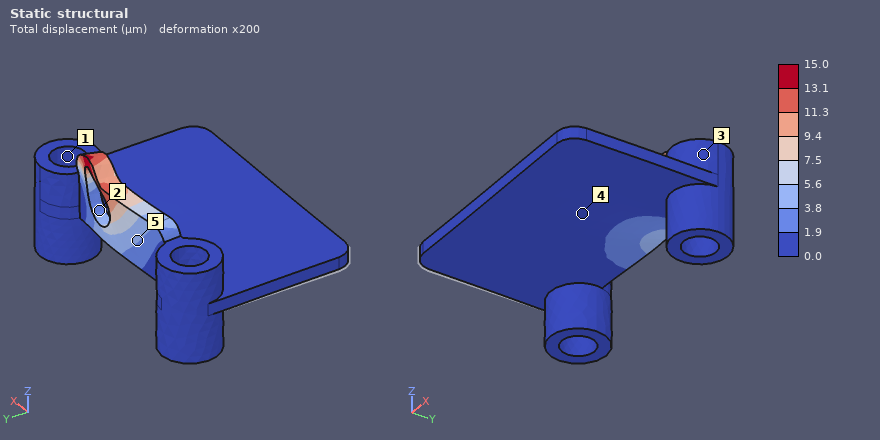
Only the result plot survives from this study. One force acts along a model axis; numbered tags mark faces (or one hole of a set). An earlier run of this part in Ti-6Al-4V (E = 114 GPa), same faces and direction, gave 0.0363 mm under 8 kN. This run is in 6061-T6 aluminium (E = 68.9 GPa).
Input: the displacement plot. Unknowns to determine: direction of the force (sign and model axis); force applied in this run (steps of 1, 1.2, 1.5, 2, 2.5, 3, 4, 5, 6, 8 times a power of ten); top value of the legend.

+X
2 kN
15.0 µm
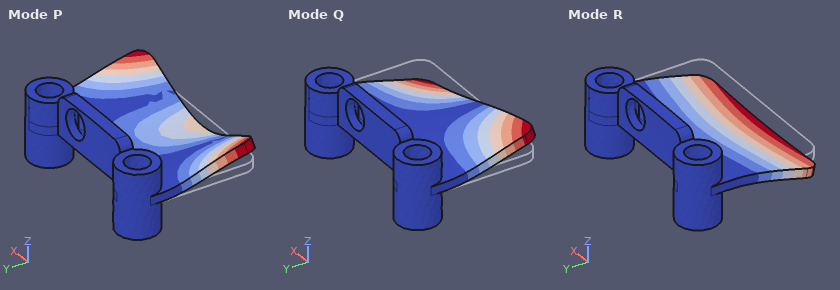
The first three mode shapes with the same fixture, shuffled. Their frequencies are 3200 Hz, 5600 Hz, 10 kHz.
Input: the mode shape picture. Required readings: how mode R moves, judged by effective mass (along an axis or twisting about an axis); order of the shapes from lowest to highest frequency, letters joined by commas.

along Z
R, Q, P
